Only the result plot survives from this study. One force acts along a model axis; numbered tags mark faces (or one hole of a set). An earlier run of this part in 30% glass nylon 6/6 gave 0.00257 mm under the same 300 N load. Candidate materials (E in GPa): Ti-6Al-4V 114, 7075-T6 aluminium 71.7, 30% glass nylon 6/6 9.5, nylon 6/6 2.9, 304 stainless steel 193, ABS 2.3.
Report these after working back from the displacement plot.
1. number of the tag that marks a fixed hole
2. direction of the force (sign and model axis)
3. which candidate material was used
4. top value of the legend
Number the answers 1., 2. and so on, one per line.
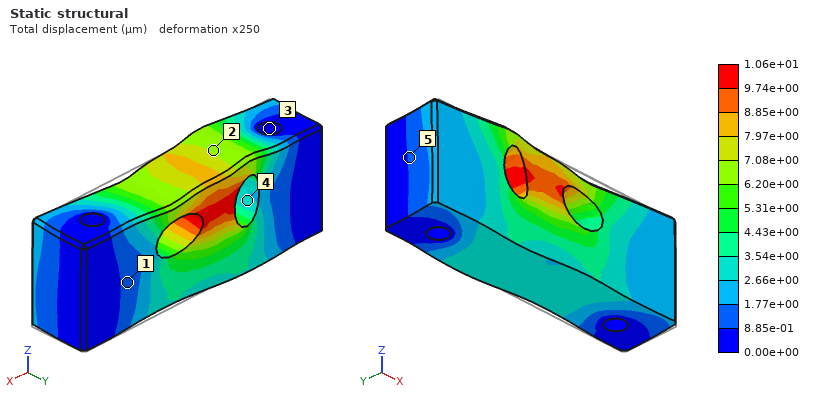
1. 3
2. -X
3. ABS
4. 1.06e+01 µm
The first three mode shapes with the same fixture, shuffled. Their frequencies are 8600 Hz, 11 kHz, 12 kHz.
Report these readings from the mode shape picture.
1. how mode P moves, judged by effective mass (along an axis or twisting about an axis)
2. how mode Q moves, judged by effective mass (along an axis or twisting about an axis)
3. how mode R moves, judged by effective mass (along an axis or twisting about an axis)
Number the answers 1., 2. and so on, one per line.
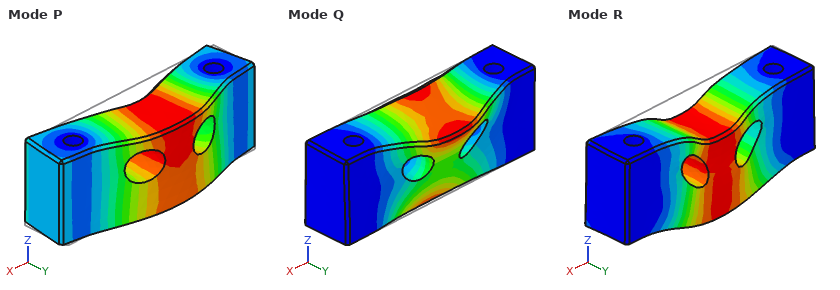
1. along Y
2. twisting about X
3. along Z
